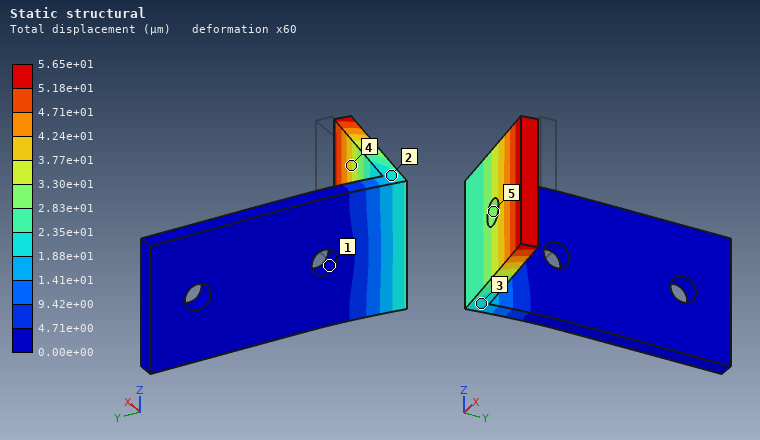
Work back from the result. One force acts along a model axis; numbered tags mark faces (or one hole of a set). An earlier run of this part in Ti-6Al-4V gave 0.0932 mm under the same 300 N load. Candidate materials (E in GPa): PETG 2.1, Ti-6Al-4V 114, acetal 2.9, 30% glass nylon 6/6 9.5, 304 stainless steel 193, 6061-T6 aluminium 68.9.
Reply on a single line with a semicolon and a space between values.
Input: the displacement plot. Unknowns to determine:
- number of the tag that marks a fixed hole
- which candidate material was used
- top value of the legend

1; 304 stainless steel; 5.65e+01 µm
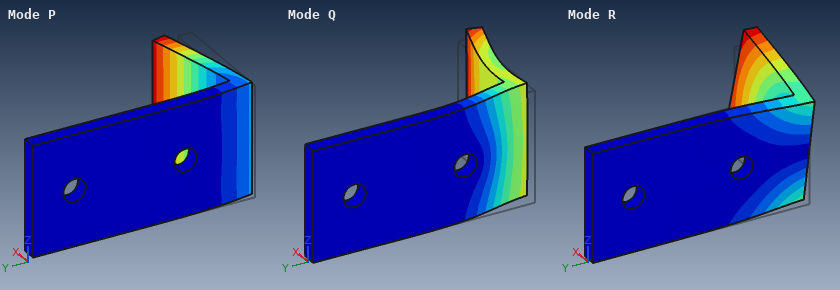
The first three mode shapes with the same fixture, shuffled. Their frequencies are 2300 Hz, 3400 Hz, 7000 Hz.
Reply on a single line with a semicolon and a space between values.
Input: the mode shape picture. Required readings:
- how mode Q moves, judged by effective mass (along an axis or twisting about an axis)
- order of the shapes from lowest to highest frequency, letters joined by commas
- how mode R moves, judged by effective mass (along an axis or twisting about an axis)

along X; P, R, Q; along Z
